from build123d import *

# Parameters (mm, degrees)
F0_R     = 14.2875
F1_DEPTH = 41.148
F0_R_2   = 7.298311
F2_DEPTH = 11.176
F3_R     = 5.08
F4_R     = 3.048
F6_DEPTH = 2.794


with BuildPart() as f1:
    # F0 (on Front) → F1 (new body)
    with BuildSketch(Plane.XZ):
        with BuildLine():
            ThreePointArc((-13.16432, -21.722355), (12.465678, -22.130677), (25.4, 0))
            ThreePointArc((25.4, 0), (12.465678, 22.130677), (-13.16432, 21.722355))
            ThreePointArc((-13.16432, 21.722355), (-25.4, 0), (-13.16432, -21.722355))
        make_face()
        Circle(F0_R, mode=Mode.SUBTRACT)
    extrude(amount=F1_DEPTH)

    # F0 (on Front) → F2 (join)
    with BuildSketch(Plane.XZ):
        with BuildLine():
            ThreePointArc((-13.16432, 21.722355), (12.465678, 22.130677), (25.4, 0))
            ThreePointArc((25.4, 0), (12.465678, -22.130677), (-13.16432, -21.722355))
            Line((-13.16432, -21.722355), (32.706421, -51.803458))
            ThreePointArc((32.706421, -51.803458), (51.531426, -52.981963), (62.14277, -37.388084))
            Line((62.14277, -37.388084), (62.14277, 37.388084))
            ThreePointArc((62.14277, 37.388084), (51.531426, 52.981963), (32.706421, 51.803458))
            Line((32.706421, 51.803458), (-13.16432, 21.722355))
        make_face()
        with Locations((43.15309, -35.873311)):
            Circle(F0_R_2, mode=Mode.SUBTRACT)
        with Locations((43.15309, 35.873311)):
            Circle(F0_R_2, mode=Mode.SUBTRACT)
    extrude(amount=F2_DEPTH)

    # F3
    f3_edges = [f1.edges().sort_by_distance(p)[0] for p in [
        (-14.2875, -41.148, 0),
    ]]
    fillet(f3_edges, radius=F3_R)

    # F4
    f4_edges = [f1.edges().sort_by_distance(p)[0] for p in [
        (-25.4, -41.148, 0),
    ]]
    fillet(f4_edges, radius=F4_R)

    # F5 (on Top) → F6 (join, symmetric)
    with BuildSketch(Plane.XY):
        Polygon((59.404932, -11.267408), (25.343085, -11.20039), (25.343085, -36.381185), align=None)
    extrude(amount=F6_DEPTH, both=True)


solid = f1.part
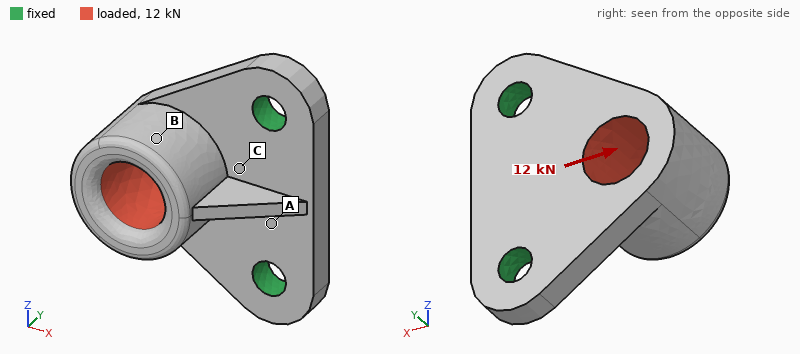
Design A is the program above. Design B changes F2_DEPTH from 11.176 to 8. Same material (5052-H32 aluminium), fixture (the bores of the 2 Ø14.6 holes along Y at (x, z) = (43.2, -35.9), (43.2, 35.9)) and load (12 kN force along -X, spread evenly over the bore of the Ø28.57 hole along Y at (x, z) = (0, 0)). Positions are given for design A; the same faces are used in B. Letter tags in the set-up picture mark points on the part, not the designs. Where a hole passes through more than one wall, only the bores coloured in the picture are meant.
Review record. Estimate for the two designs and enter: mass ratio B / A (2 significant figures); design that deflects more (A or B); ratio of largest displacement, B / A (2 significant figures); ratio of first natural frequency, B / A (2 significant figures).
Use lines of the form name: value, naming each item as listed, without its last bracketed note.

mass ratio B / A: 0.87
design that deflects more: B
ratio of largest displacement, B / A: 2.6
ratio of first natural frequency, B / A: 0.65
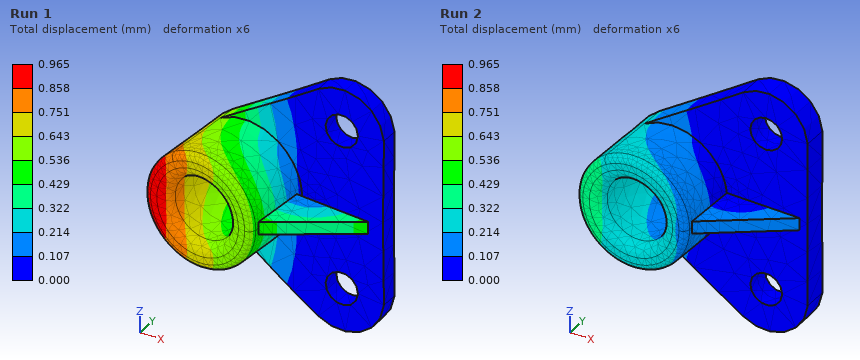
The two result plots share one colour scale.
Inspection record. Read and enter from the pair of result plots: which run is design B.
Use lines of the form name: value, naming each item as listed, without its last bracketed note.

which run is design B: Run 1
